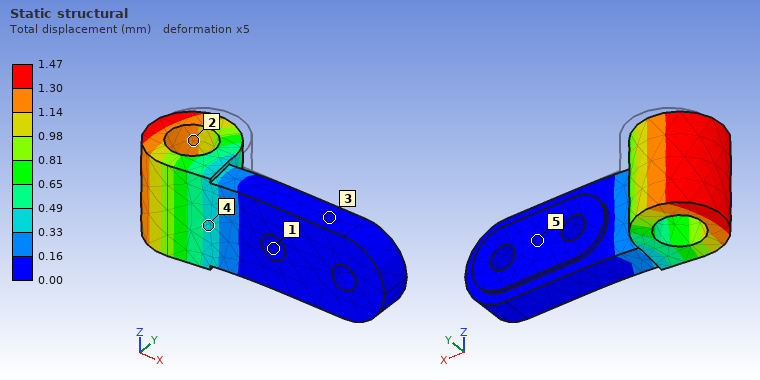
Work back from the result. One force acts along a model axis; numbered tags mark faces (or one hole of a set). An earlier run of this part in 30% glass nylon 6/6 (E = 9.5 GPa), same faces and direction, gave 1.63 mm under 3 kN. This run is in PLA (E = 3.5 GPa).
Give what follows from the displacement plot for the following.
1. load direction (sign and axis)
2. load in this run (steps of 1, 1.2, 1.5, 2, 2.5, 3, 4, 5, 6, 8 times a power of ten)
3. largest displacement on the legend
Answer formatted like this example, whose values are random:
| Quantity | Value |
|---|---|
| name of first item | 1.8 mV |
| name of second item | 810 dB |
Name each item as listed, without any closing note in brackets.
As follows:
| Quantity | Value |
|---|---|
| load direction | -Y |
| load in this run | 1 kN |
| largest displacement on the legend | 1.47 mm |
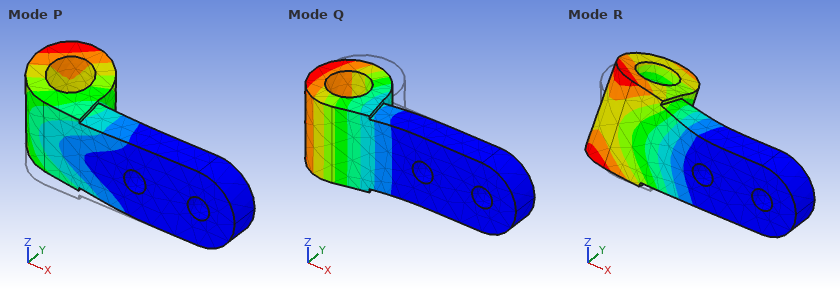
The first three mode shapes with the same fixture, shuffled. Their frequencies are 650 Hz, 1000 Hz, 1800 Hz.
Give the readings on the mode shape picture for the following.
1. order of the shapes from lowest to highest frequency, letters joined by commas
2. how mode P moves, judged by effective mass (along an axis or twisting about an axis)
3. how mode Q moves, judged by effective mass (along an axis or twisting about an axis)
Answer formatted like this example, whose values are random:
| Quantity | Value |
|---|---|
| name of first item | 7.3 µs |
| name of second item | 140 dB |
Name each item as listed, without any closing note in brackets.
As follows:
| Quantity | Value |
|---|---|
| order of the shapes from lowest to highest frequency, letters joined by commas | Q, P, R |
| how mode P moves, judged by effective mass | along Z |
| how mode Q moves, judged by effective mass | along Y |
